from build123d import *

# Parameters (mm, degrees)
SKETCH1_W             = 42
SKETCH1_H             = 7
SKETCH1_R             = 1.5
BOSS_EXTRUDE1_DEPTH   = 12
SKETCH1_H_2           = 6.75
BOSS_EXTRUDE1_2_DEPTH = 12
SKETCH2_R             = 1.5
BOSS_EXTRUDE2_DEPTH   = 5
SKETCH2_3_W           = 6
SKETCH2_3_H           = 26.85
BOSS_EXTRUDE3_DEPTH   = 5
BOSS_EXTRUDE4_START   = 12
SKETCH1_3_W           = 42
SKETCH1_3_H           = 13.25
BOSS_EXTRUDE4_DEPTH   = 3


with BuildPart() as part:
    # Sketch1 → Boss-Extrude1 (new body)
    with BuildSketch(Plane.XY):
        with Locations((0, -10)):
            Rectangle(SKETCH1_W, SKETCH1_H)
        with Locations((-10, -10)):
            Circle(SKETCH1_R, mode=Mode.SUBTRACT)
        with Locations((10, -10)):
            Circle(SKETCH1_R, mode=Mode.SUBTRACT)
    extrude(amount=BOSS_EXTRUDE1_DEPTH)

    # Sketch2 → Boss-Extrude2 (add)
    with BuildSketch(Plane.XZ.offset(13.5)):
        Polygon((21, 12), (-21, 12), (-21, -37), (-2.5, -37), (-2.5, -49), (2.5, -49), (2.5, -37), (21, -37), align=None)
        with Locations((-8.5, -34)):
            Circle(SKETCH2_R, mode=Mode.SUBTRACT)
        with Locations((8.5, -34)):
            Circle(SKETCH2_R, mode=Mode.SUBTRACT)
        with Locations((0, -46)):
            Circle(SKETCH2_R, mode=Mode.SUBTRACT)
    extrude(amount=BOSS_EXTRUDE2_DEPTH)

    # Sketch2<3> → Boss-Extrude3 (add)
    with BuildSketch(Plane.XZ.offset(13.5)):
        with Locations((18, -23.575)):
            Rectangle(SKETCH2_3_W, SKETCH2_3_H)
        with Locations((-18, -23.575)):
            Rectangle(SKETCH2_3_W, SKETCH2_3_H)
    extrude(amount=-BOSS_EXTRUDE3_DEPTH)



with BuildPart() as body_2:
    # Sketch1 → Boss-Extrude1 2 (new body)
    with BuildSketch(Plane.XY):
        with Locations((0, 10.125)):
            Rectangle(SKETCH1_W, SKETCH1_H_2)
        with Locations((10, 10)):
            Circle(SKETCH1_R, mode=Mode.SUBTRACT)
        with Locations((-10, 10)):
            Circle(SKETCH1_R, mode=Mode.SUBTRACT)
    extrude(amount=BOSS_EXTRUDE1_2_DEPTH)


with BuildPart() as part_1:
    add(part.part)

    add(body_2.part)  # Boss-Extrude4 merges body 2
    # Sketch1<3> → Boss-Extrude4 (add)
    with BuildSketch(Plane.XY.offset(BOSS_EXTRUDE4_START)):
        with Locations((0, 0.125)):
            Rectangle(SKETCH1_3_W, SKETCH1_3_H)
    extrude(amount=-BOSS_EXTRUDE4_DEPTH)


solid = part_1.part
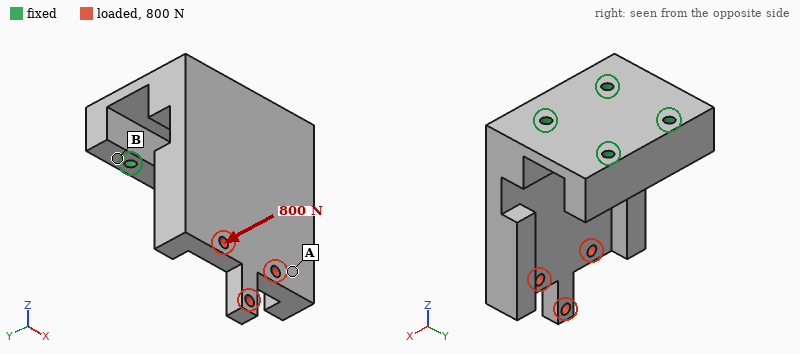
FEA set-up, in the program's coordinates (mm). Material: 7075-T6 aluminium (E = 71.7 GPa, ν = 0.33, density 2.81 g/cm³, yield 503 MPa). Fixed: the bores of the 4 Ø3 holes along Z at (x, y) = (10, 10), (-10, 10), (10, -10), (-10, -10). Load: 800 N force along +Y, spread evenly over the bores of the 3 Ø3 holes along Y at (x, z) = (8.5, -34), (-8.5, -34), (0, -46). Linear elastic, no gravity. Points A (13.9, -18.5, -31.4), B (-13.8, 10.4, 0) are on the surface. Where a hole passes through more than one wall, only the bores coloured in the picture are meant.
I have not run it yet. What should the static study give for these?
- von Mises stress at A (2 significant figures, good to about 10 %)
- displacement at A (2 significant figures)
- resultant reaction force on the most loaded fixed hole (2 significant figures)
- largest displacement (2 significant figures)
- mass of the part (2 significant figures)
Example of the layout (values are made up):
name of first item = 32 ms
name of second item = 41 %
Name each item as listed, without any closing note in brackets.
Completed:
von Mises stress at A = 35 MPa
displacement at A = 0.38 mm
resultant reaction force on the most loaded fixed hole = 690 N
largest displacement = 0.78 mm
mass of the part = 57 g
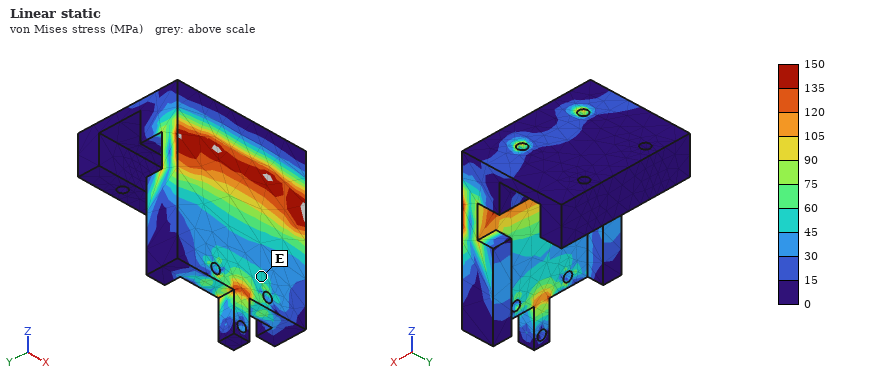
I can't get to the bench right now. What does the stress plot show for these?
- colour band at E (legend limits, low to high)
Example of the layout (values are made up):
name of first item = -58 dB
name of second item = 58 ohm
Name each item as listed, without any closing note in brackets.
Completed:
colour band at E = 45 to 60 MPa
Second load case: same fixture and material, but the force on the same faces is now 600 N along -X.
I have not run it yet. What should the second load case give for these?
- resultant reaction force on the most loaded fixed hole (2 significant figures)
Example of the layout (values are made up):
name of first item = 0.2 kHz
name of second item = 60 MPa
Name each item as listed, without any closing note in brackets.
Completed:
resultant reaction force on the most loaded fixed hole = 960 N
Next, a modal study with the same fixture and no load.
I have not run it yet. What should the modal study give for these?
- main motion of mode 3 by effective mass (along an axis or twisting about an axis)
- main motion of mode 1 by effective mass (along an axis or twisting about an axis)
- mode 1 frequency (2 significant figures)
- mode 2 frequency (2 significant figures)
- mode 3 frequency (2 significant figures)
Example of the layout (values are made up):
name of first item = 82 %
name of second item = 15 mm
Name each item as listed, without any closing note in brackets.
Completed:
main motion of mode 3 by effective mass = along X
main motion of mode 1 by effective mass = along Y
mode 1 frequency = 2200 Hz
mode 2 frequency = 4700 Hz
mode 3 frequency = 8200 Hz
